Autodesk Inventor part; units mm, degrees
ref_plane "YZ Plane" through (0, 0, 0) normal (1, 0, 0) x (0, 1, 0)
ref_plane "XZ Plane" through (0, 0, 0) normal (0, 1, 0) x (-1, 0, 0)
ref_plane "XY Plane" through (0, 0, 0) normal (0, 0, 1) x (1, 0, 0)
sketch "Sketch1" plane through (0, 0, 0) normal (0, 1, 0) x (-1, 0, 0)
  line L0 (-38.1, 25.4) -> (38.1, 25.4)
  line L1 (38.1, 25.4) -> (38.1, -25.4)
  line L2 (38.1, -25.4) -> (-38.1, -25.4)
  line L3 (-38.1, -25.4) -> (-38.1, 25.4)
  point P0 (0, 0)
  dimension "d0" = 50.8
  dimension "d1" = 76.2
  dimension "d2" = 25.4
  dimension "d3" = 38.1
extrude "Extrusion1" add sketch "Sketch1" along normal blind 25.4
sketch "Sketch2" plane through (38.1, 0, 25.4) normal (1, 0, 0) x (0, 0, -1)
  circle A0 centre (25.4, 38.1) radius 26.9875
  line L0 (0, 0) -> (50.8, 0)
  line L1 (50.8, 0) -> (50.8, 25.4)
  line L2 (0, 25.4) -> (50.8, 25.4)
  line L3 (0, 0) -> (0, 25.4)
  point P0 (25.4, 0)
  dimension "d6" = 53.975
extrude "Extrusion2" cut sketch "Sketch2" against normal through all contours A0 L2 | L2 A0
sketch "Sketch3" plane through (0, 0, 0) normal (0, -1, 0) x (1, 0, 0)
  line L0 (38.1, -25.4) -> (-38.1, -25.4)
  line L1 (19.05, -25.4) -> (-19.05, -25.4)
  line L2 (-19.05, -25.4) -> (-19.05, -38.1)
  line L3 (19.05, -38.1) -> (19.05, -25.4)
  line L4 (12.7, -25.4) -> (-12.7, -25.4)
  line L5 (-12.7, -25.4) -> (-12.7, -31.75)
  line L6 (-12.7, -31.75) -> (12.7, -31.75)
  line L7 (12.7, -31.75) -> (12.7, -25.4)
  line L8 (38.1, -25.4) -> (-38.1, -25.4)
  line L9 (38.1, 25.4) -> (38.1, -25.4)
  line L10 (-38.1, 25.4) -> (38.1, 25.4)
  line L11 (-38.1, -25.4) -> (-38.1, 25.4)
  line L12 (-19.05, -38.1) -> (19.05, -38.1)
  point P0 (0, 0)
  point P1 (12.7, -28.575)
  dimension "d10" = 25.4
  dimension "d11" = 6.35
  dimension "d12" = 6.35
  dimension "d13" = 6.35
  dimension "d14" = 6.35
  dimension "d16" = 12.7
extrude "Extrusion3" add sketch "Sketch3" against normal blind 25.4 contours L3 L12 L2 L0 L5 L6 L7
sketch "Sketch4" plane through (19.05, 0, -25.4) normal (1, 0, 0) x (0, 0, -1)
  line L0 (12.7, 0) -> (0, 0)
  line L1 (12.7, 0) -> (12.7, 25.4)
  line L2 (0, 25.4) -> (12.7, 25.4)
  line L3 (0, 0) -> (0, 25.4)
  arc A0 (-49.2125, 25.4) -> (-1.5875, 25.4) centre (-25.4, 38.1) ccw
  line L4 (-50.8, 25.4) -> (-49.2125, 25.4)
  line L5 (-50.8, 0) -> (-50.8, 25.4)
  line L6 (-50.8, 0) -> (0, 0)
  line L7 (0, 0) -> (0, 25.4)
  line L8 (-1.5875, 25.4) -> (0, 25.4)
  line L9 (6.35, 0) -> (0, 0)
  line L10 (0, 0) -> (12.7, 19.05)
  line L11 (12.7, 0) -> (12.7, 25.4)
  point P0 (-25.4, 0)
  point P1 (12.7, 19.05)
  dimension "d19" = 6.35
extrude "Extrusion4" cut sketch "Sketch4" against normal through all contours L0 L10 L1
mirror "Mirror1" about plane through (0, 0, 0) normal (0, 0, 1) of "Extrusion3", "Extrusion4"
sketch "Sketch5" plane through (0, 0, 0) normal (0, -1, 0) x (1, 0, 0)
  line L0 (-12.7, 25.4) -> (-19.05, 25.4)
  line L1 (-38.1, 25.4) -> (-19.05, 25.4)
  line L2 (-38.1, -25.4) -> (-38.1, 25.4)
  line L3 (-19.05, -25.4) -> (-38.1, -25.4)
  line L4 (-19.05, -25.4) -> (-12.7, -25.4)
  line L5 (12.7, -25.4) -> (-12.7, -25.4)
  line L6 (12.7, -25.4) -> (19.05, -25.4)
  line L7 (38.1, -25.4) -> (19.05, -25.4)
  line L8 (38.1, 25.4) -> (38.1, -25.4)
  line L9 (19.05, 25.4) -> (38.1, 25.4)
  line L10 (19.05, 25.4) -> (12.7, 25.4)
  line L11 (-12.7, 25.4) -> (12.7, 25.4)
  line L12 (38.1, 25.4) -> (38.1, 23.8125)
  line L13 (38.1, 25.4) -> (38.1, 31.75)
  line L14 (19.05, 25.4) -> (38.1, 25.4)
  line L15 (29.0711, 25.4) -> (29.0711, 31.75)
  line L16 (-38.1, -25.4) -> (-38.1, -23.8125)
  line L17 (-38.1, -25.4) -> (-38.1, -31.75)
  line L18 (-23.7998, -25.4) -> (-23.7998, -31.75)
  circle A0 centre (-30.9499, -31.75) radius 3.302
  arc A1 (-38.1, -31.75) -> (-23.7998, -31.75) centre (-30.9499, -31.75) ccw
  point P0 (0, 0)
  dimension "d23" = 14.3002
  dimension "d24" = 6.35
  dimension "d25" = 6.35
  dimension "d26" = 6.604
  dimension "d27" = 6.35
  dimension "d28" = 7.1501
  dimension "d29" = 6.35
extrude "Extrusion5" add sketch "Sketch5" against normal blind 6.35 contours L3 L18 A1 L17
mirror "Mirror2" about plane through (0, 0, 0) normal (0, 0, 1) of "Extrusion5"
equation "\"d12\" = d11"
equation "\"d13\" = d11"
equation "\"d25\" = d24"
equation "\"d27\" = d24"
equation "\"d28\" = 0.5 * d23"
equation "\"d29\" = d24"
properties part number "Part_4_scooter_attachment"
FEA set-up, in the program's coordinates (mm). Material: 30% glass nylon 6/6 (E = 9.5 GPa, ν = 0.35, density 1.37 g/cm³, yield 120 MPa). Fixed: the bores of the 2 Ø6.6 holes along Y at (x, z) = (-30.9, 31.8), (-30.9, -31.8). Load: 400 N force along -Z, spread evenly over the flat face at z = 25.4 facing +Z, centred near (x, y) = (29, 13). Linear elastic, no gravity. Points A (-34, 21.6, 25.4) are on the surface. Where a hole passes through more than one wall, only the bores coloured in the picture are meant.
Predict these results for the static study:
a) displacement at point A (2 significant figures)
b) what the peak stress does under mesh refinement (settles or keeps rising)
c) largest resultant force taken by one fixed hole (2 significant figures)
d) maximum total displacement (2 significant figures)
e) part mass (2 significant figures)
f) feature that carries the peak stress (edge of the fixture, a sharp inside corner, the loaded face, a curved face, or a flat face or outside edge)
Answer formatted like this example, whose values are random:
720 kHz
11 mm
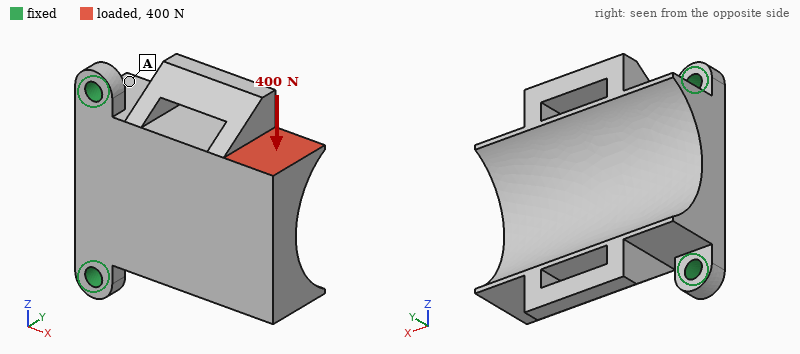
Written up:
16 µm
keeps rising
470 N
99 µm
98 g
edge of the fixture
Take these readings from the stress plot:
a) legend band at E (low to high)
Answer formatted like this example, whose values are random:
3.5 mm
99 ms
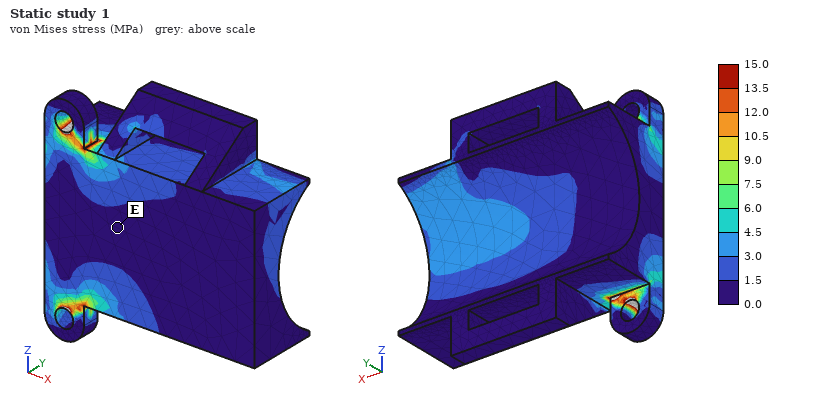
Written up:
0.0 to 1.5 MPa
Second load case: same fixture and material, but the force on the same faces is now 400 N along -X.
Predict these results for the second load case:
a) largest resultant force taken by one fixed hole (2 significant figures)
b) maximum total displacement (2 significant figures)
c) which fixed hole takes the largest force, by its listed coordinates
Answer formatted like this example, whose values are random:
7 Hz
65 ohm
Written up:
380 N
0.26 mm
(-30.9, 31.8)
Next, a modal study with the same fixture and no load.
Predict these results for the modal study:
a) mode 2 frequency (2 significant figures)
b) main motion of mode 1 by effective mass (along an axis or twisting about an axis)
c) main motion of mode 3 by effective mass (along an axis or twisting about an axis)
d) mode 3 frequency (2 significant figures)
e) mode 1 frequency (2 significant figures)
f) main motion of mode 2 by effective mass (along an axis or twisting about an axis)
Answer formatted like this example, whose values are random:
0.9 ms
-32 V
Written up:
2000 Hz
along Y
along Z
2100 Hz
440 Hz
twisting about X
